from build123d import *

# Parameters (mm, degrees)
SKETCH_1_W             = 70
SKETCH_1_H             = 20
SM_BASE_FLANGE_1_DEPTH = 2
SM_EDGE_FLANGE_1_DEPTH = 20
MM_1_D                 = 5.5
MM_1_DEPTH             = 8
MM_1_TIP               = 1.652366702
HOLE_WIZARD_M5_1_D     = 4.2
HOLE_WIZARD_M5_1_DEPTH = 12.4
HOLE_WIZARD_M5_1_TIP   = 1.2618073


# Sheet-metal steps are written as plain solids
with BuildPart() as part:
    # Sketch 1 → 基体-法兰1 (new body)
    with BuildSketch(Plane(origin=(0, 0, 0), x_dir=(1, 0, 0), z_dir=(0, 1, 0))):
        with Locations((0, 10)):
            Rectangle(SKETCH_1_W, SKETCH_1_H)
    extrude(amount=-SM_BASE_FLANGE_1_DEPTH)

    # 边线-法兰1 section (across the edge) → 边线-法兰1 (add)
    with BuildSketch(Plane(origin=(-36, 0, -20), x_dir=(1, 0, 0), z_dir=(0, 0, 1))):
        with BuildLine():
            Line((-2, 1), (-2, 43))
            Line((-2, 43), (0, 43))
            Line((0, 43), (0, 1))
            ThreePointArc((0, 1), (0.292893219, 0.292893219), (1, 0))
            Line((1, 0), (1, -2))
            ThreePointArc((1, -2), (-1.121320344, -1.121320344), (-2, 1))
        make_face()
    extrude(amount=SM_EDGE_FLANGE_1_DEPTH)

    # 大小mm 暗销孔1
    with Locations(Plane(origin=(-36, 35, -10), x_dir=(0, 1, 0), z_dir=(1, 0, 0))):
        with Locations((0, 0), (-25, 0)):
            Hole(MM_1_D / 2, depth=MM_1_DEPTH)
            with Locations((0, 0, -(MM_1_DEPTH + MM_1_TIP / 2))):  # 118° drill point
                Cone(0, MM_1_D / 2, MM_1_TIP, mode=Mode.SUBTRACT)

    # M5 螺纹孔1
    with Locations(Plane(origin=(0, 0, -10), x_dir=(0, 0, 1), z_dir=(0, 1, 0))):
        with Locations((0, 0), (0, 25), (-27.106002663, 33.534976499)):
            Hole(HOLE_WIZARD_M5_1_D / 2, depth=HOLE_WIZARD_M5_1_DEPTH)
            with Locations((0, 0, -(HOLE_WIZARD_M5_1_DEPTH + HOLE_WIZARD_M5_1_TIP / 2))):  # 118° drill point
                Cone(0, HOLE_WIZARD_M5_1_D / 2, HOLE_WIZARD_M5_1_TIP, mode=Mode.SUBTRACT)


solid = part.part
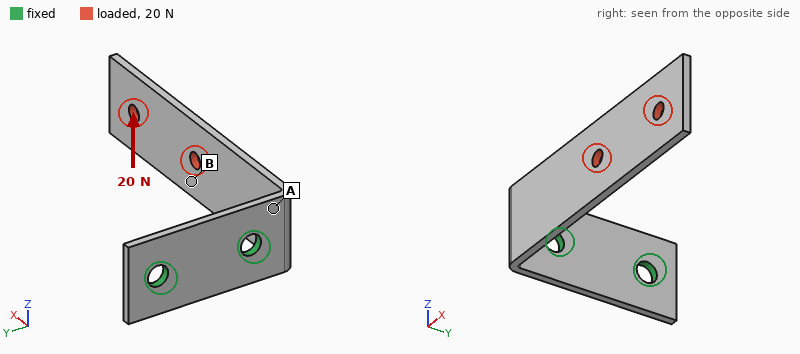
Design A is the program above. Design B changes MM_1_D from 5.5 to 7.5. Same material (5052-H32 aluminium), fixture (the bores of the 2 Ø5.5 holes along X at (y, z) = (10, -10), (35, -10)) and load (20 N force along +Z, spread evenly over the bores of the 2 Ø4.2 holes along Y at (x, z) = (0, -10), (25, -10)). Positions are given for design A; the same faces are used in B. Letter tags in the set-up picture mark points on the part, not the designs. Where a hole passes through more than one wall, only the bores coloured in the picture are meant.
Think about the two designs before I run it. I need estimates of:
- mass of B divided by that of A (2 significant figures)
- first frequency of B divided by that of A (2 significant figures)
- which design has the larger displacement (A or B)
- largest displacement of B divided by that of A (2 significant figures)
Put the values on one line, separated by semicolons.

0.98; 1.0; A; 0.79
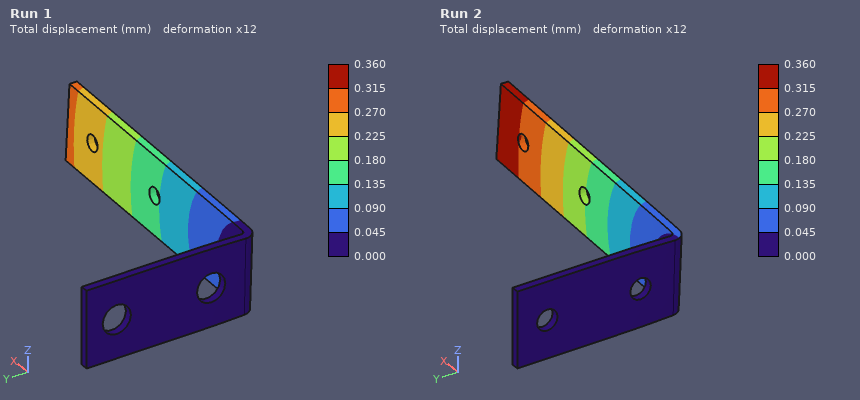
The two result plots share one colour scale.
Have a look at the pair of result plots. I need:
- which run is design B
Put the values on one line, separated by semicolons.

Run 1
